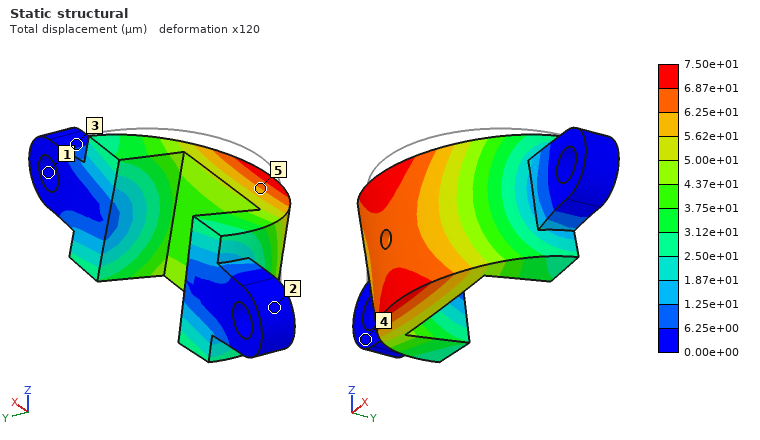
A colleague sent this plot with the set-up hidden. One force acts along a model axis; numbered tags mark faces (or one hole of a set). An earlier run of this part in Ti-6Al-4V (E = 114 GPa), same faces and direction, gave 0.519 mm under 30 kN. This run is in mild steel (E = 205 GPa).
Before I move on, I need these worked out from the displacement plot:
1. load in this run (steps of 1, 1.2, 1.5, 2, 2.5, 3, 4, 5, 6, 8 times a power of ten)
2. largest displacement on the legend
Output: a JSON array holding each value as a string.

["8 kN", "7.50e+01 µm"]
